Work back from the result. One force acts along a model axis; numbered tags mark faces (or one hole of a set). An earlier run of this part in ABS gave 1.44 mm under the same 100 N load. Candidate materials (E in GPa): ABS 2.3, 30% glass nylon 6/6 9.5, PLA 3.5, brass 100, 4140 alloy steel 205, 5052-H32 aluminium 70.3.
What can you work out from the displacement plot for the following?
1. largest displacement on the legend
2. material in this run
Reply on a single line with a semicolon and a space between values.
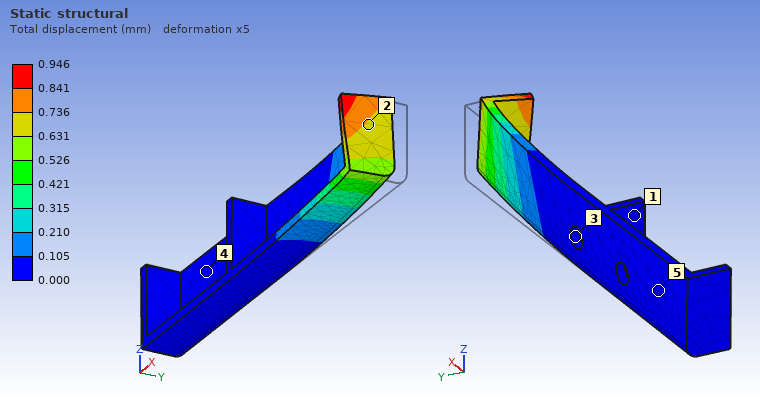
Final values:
0.946 mm; PLA
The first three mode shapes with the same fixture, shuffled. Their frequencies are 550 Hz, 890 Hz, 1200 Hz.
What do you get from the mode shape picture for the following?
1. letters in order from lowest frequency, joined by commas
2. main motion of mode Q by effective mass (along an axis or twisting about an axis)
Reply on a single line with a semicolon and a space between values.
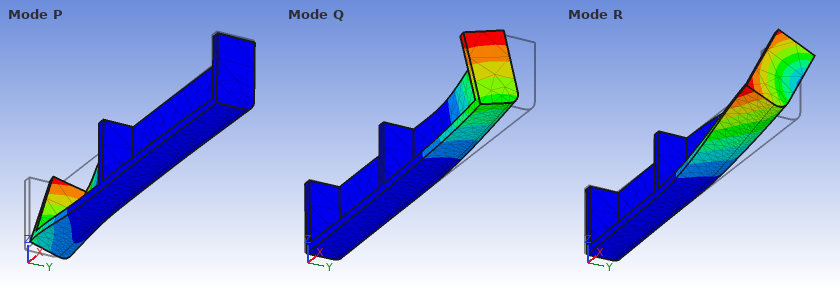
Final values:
Q, R, P; along Y
